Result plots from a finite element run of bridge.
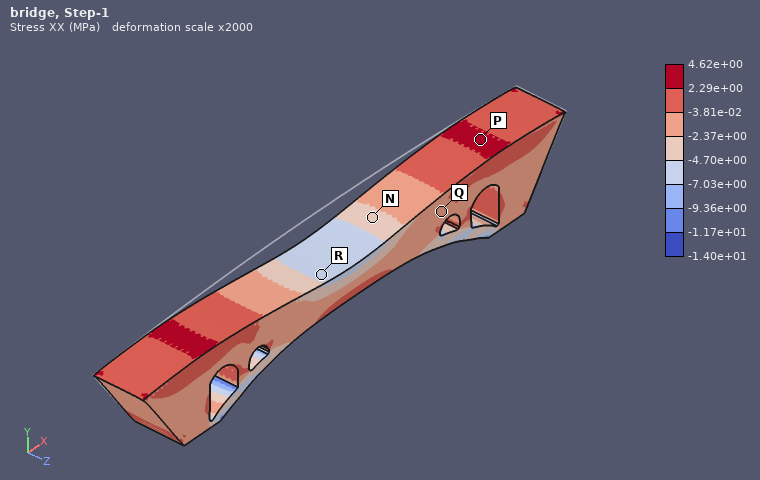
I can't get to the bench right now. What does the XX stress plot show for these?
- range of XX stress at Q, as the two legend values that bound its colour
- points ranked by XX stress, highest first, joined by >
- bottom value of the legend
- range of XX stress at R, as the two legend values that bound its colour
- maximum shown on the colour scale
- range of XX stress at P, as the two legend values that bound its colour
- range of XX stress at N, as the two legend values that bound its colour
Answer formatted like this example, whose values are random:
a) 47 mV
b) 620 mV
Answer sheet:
a) -2.37e+00 to -3.81e-02 MPa
b) P > Q > N > R
c) -1.40e+01 MPa
d) -7.03e+00 to -4.70e+00 MPa
e) 4.62e+00 MPa
f) 2.29e+00 to 4.62e+00 MPa
g) -4.70e+00 to -2.37e+00 MPa
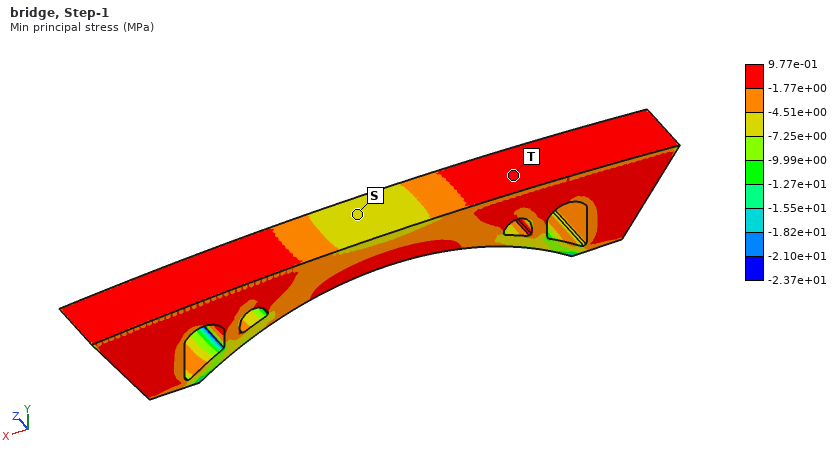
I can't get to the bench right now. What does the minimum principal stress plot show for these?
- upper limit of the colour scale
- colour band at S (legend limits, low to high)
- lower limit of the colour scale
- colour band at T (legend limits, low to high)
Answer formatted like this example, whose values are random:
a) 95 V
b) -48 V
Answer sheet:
a) 9.77e-01 MPa
b) -7.25e+00 to -4.51e+00 MPa
c) -2.37e+01 MPa
d) -1.77e+00 to 9.77e-01 MPa
